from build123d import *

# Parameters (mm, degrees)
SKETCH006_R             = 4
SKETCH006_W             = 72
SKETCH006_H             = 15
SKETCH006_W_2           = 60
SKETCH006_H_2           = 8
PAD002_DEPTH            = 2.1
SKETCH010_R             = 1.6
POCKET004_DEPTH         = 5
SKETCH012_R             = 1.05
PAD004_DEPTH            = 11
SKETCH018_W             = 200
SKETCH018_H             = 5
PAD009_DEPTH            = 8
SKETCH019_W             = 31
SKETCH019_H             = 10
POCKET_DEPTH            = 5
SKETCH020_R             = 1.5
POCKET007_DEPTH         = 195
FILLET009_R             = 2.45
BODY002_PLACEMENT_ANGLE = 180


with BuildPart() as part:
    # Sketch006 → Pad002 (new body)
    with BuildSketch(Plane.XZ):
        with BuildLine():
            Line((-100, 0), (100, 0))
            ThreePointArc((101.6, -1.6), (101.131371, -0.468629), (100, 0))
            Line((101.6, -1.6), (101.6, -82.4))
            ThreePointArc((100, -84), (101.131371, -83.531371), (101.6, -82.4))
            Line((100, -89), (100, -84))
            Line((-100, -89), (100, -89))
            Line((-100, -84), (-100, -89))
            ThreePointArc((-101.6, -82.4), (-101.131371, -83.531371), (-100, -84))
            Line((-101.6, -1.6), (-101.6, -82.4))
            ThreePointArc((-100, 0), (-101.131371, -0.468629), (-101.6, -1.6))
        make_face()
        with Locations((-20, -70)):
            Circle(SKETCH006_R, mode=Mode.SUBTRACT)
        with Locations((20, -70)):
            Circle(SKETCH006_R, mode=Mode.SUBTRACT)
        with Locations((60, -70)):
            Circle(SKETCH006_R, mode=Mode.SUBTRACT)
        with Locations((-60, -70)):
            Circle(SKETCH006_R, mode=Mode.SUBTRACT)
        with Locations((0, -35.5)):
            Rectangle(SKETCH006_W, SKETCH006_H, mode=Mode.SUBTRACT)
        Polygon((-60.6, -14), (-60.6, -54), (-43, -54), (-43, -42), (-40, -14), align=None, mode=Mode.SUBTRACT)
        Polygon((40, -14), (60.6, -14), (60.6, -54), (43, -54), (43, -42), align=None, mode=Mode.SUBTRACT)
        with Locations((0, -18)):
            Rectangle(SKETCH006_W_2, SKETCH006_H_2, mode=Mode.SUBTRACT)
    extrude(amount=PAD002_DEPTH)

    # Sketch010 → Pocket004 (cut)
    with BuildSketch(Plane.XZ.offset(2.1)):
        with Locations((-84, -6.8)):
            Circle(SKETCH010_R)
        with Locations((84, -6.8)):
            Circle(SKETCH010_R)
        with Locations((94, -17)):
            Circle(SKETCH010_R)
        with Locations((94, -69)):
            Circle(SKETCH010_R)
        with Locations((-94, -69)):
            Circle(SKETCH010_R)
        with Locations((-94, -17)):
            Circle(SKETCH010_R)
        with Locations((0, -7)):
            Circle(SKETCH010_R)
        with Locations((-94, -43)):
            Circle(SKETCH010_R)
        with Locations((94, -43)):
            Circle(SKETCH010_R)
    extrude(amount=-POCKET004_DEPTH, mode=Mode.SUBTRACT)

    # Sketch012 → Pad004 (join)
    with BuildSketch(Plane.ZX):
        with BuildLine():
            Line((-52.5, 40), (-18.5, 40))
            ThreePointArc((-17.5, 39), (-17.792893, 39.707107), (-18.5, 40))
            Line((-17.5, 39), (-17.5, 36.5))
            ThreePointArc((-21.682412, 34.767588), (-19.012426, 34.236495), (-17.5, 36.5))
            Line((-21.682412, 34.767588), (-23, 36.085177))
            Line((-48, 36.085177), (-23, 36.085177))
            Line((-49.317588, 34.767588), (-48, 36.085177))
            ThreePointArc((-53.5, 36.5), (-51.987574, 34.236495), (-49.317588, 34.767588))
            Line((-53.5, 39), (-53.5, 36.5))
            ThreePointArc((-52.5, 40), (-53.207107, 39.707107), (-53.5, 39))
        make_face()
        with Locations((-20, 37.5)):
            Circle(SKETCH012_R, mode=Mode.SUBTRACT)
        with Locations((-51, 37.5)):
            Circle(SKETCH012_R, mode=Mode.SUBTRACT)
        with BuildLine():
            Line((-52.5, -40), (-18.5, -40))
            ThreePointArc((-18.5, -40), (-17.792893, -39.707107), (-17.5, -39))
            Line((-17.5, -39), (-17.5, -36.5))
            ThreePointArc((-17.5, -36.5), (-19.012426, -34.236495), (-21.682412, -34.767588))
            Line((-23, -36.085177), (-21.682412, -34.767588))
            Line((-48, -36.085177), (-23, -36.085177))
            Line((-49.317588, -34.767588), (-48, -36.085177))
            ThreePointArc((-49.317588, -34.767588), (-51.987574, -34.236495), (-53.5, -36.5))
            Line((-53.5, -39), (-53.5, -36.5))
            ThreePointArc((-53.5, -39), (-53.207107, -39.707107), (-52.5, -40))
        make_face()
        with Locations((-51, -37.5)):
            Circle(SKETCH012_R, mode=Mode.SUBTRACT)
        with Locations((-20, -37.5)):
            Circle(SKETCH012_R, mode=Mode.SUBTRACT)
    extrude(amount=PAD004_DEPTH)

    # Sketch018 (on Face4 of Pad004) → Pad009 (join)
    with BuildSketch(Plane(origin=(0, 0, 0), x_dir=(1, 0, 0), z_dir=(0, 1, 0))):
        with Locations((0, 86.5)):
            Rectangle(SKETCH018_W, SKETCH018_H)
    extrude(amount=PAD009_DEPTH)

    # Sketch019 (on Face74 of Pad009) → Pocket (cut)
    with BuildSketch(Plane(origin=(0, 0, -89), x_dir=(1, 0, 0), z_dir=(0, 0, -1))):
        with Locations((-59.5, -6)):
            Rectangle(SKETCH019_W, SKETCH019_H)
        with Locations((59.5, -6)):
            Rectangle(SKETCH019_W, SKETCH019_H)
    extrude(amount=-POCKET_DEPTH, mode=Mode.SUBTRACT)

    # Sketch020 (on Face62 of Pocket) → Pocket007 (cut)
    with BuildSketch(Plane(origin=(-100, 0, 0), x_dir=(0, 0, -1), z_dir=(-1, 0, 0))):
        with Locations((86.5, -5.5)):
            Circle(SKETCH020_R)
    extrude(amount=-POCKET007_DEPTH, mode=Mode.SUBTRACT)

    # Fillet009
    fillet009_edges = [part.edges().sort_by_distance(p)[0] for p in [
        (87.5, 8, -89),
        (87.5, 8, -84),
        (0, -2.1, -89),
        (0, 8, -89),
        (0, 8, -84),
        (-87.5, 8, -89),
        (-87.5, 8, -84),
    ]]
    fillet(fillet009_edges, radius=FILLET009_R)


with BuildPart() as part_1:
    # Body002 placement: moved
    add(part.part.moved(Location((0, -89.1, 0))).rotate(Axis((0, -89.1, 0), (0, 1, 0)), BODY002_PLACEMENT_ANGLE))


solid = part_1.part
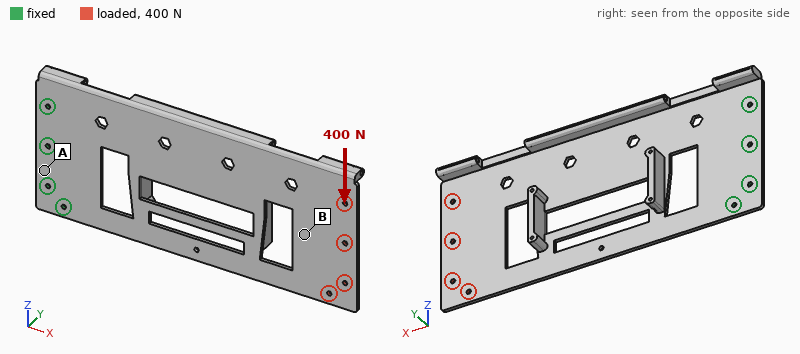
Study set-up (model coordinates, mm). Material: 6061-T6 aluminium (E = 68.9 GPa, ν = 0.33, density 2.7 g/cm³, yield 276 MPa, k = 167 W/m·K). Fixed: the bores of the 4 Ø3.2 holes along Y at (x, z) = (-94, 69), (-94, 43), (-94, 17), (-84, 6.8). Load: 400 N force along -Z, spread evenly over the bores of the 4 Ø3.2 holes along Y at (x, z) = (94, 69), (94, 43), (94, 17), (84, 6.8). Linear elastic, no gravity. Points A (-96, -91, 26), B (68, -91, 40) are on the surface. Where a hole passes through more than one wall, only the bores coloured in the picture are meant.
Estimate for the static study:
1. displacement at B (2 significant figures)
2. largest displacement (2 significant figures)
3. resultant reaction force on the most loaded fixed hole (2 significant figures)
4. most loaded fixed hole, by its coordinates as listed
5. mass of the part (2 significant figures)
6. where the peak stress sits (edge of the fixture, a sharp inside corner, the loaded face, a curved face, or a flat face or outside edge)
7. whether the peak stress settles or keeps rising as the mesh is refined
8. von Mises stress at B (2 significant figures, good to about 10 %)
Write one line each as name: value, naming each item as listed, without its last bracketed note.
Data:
displacement at B: 0.59 mm
largest displacement: 0.75 mm
resultant reaction force on the most loaded fixed hole: 1.2 kN
most loaded fixed hole, by its coordinates as listed: (-94, 69)
mass of the part: 100 g
where the peak stress sits: edge of the fixture
whether the peak stress settles or keeps rising as the mesh is refined: keeps rising
von Mises stress at B: 11 MPa
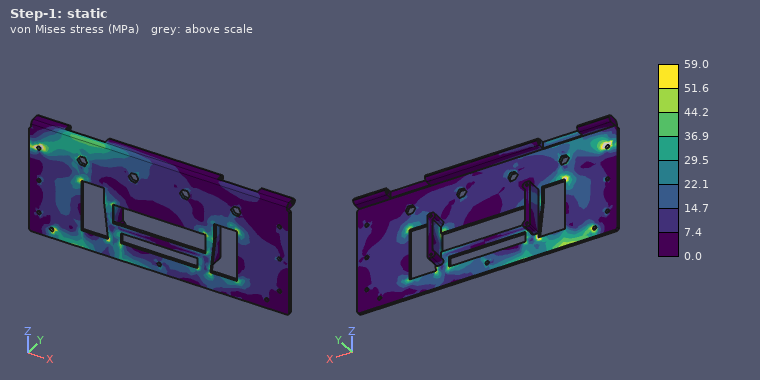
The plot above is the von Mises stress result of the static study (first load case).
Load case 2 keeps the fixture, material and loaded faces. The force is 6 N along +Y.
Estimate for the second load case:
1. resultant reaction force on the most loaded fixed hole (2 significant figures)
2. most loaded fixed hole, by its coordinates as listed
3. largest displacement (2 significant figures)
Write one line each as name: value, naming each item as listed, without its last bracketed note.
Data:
resultant reaction force on the most loaded fixed hole: 25 N
most loaded fixed hole, by its coordinates as listed: (-94, 69)
largest displacement: 2.5 mm
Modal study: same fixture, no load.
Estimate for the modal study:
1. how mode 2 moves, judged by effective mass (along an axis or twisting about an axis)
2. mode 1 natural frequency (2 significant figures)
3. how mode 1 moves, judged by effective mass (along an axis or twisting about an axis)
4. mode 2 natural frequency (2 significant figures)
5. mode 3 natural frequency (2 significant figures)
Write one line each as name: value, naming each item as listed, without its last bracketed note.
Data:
how mode 2 moves, judged by effective mass: twisting about X
mode 1 natural frequency: 47 Hz
how mode 1 moves, judged by effective mass: along Y
mode 2 natural frequency: 210 Hz
mode 3 natural frequency: 360 Hz
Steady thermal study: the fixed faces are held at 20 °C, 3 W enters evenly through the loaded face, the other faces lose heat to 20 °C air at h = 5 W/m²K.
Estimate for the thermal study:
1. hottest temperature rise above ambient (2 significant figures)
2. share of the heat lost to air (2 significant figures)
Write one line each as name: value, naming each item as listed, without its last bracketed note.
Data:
hottest temperature rise above ambient: 18 K
share of the heat lost to air: 47 %
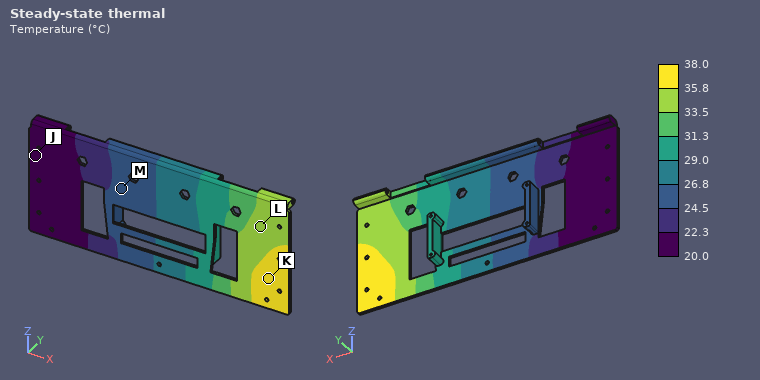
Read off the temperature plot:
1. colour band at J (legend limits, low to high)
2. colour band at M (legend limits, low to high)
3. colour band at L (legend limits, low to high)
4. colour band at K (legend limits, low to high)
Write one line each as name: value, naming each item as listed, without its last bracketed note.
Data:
colour band at J: 20.0 to 22.3 °C
colour band at M: 24.5 to 26.8 °C
colour band at L: 33.5 to 35.8 °C
colour band at K: 35.8 to 38.0 °C
